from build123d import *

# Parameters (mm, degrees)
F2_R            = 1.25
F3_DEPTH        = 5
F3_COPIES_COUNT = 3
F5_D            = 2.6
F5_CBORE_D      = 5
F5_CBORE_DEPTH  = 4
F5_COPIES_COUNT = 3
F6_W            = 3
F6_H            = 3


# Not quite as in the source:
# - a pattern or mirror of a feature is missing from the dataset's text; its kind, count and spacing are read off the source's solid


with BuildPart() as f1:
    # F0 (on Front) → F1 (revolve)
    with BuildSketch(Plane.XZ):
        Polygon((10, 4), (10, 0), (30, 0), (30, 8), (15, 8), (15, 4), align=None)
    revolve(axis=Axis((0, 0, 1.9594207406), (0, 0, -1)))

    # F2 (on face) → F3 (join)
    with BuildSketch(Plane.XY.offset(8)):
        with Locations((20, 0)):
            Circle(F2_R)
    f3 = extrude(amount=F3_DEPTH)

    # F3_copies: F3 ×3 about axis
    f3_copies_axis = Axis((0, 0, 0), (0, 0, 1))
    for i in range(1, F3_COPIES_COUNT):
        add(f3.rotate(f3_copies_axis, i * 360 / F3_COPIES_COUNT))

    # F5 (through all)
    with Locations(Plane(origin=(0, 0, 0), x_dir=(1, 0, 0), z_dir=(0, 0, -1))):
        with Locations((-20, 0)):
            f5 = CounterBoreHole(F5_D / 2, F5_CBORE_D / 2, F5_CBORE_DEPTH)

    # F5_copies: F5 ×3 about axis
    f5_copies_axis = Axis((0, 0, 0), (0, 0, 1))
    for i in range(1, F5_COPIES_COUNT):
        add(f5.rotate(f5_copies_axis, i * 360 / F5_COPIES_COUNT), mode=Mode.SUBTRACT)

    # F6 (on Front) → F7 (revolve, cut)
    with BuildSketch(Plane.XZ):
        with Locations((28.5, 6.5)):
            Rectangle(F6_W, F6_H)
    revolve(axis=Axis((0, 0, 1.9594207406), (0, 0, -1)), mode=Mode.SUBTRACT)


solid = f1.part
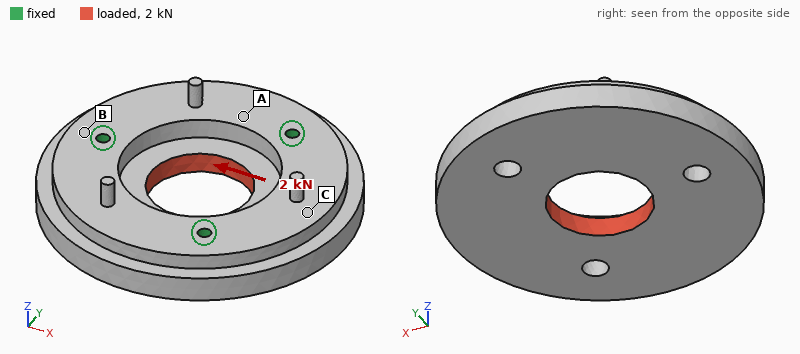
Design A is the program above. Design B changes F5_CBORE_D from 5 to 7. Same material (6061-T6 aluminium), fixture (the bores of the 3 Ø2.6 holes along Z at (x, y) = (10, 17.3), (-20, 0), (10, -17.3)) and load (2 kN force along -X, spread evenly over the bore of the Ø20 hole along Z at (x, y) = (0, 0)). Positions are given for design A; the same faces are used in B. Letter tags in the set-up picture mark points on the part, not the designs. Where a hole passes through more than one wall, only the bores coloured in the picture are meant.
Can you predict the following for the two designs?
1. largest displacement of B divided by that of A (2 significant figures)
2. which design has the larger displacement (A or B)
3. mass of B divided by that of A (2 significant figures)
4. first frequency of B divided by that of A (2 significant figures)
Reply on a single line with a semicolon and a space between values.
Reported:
1.1; B; 0.99; 0.97
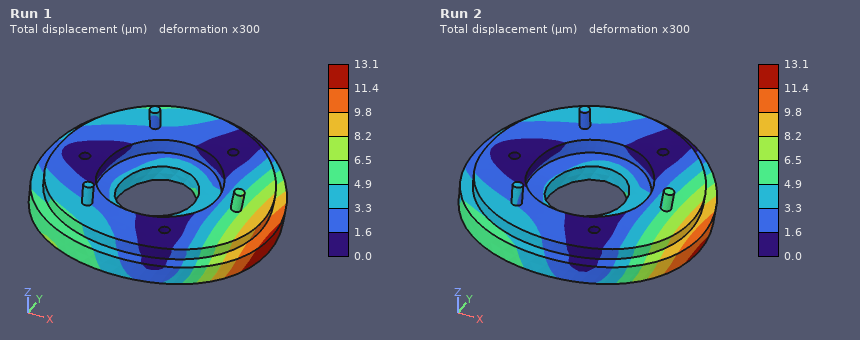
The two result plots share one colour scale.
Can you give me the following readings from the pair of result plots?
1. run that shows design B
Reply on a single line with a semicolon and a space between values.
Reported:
Run 1
